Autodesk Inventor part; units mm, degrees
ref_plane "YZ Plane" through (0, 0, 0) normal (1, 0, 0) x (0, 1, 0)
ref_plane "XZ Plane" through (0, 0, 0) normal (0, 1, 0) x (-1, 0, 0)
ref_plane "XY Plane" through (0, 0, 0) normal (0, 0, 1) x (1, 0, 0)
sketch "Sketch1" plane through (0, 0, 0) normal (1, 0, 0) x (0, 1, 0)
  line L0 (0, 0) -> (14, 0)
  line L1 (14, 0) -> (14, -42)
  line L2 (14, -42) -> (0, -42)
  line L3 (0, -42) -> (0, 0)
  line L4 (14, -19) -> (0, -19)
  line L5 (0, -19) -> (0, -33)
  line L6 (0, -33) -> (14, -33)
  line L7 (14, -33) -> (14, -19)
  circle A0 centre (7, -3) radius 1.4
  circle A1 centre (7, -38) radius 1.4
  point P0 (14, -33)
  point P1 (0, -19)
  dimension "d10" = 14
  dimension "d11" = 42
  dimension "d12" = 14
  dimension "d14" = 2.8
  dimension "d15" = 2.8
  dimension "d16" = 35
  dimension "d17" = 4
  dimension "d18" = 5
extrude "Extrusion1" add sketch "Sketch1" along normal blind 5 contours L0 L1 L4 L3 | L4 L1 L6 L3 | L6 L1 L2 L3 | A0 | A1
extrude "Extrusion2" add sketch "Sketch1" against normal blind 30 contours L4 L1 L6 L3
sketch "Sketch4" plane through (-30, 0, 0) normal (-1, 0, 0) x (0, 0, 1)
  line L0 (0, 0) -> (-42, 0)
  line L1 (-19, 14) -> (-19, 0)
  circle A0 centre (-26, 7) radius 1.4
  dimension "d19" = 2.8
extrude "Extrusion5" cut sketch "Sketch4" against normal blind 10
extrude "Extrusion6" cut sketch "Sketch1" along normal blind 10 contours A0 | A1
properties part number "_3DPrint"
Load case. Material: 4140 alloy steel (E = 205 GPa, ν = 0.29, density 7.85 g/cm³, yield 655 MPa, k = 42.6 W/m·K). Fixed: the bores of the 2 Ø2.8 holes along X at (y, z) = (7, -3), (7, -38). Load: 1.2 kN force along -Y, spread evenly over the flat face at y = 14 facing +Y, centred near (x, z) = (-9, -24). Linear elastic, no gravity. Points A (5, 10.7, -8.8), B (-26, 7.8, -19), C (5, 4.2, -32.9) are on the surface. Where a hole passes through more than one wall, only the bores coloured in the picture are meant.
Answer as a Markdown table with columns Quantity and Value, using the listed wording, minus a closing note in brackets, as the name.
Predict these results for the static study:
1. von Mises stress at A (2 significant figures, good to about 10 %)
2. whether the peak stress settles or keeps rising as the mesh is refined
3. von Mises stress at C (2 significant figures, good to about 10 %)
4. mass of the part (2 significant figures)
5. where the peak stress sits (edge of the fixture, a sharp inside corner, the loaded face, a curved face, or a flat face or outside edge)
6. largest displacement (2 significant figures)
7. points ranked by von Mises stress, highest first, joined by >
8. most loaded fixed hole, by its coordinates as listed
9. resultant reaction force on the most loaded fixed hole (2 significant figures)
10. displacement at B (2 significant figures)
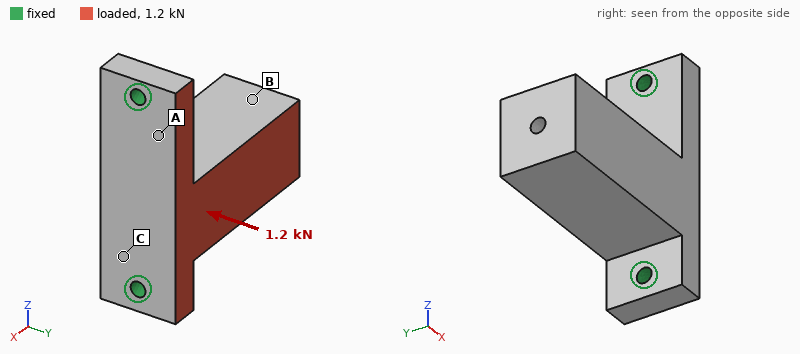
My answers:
| Quantity | Value |
|---|---|
| von Mises stress at A | 48 MPa |
| whether the peak stress settles or keeps rising as the mesh is refined | keeps rising |
| von Mises stress at C | 72 MPa |
| mass of the part | 68 g |
| where the peak stress sits | edge of the fixture |
| largest displacement | 68 µm |
| points ranked by von Mises stress, highest first, joined by > | C > A > B |
| most loaded fixed hole, by its coordinates as listed | (7, -38) |
| resultant reaction force on the most loaded fixed hole | 760 N |
| displacement at B | 59 µm |
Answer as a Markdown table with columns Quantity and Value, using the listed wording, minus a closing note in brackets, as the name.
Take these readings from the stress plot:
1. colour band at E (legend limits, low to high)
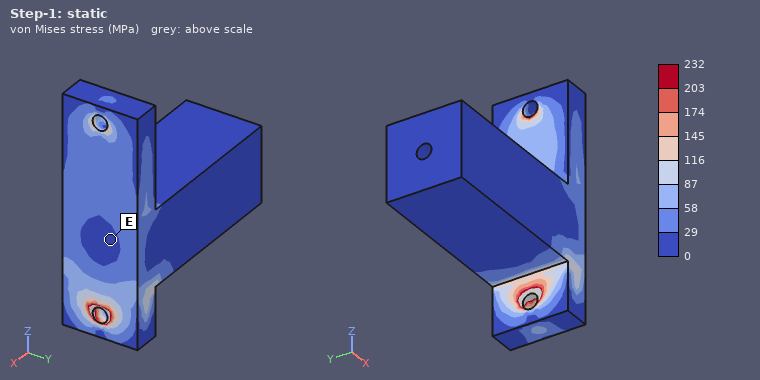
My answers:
| Quantity | Value |
|---|---|
| colour band at E | 0 to 29 MPa |
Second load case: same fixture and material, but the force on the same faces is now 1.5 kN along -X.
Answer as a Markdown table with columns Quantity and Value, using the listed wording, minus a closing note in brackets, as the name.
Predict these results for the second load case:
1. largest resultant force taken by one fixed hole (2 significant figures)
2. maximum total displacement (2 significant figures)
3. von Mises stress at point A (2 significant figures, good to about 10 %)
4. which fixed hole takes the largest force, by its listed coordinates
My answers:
| Quantity | Value |
|---|---|
| largest resultant force taken by one fixed hole | 940 N |
| maximum total displacement | 47 µm |
| von Mises stress at point A | 44 MPa |
| which fixed hole takes the largest force, by its listed coordinates | (7, -38) |
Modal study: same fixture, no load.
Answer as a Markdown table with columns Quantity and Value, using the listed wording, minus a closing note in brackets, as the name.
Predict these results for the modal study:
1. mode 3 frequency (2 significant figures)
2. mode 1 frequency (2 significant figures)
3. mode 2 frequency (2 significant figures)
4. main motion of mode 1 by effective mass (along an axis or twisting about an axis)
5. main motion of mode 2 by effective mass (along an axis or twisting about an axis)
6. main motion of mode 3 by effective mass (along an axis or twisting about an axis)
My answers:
| Quantity | Value |
|---|---|
| mode 3 frequency | 12 kHz |
| mode 1 frequency | 3100 Hz |
| mode 2 frequency | 5100 Hz |
| main motion of mode 1 by effective mass | along Y |
| main motion of mode 2 by effective mass | along Z |
| main motion of mode 3 by effective mass | along X |
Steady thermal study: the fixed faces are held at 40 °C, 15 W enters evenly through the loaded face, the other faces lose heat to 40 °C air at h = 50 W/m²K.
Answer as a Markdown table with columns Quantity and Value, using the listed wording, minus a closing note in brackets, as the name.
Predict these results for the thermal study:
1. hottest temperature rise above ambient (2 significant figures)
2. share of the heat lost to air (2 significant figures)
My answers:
| Quantity | Value |
|---|---|
| hottest temperature rise above ambient | 37 K |
| share of the heat lost to air | 20 % |
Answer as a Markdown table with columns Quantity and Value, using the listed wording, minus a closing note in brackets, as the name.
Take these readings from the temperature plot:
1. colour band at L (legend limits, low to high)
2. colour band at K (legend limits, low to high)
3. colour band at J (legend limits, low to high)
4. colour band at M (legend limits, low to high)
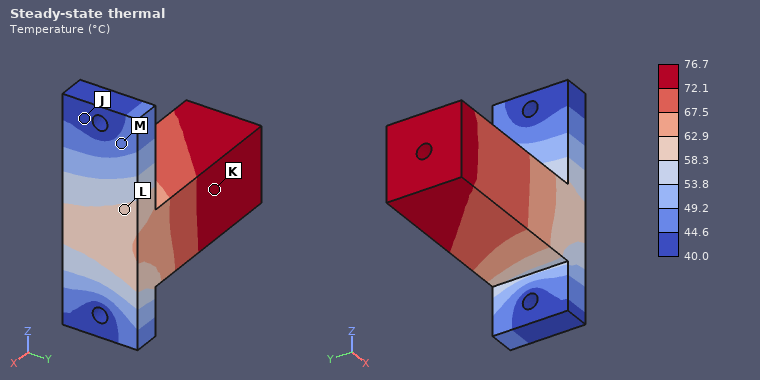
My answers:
| Quantity | Value |
|---|---|
| colour band at L | 58.3 to 62.9 °C |
| colour band at K | 72.1 to 76.7 °C |
| colour band at J | 40.0 to 44.6 °C |
| colour band at M | 44.6 to 49.2 °C |
